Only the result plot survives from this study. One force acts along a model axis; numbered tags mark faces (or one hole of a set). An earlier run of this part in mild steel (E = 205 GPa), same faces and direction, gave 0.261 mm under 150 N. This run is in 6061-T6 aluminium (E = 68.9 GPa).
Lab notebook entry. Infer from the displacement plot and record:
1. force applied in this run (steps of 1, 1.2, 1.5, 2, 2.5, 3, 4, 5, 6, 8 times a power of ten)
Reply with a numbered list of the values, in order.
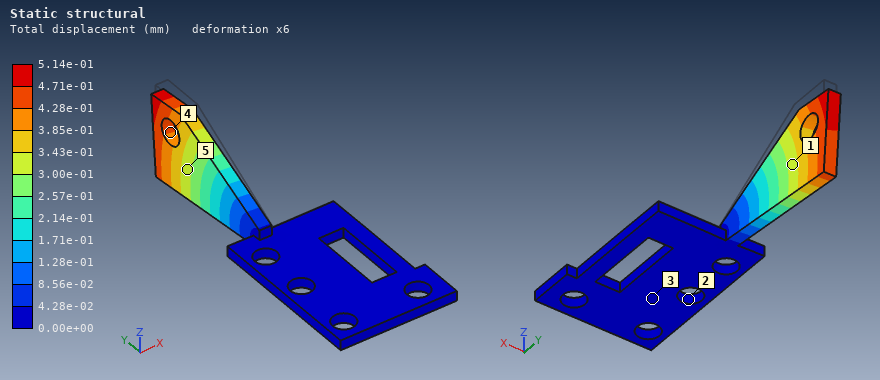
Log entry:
1. 100 N
